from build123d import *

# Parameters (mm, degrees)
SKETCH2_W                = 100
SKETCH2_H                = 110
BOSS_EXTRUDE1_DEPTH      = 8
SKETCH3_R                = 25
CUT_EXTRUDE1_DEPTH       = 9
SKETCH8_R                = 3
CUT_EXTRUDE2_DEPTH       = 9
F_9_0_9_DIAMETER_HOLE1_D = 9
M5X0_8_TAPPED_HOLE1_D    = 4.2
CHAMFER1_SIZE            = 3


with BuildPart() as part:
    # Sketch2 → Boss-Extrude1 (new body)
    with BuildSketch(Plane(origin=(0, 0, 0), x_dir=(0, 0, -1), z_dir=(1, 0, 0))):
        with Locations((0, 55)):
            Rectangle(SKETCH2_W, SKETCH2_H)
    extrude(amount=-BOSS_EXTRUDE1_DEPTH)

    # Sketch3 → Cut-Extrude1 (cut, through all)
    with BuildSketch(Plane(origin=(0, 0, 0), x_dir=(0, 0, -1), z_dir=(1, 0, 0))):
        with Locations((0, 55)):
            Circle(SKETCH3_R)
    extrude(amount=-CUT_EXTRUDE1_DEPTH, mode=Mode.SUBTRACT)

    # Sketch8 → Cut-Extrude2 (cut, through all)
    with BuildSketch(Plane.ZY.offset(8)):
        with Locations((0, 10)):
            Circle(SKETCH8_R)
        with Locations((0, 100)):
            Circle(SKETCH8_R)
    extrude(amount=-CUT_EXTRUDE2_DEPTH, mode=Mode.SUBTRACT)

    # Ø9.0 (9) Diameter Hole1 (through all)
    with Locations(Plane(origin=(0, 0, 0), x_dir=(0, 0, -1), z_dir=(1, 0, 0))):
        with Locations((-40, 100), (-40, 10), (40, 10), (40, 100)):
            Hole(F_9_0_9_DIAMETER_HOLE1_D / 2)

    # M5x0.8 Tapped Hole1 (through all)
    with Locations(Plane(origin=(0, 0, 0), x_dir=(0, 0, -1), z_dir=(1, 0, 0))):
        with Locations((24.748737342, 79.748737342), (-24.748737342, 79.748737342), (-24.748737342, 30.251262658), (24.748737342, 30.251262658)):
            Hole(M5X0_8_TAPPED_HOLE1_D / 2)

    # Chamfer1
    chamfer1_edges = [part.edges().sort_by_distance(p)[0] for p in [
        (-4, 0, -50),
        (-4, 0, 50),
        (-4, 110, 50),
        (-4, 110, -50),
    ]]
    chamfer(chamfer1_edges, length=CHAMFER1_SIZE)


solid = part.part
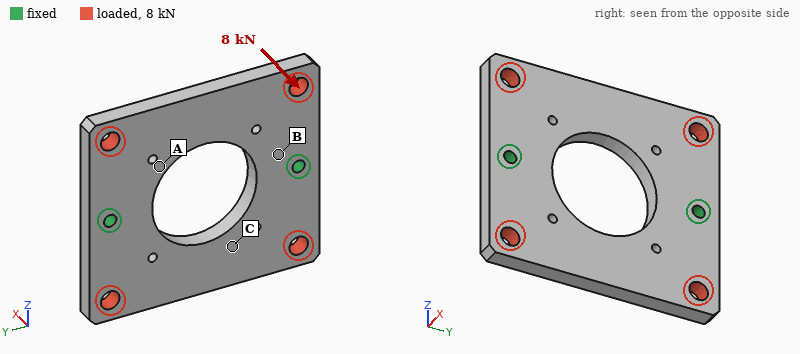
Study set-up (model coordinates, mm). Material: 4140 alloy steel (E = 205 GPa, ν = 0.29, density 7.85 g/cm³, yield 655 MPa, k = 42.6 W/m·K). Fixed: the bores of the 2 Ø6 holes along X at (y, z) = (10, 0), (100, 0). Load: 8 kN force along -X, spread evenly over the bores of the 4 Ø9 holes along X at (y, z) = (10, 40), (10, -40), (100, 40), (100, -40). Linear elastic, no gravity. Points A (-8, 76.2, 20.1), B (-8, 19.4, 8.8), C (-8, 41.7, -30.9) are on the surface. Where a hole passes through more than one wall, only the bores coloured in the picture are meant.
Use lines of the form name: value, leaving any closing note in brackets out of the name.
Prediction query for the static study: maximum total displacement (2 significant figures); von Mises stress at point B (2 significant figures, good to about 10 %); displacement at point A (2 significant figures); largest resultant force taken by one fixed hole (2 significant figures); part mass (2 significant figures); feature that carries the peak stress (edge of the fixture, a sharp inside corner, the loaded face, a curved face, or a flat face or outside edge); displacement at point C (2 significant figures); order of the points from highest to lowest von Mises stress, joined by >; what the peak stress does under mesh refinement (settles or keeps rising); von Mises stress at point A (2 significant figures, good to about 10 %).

maximum total displacement: 0.20 mm
von Mises stress at point B: 170 MPa
displacement at point A: 0.044 mm
largest resultant force taken by one fixed hole: 4.0 kN
part mass: 540 g
feature that carries the peak stress: edge of the fixture
displacement at point C: 0.087 mm
order of the points from highest to lowest von Mises stress, joined by >: B > A > C
what the peak stress does under mesh refinement: keeps rising
von Mises stress at point A: 81 MPa
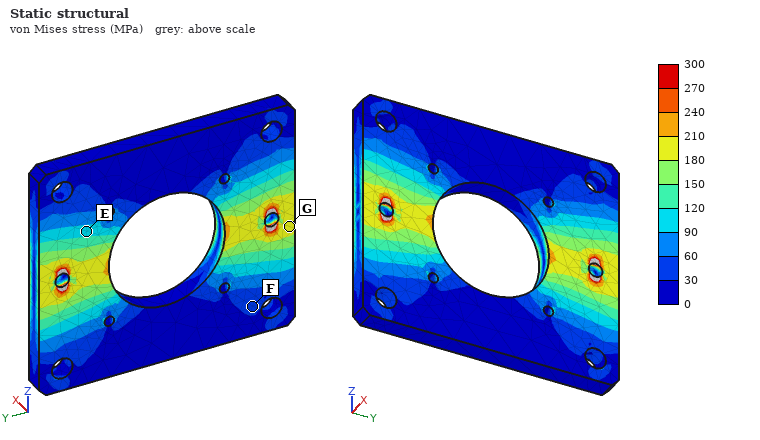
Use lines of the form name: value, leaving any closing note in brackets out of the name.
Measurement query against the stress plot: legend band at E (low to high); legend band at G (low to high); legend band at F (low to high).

legend band at E: 90 to 120 MPa
legend band at G: 180 to 210 MPa
legend band at F: 30 to 60 MPa
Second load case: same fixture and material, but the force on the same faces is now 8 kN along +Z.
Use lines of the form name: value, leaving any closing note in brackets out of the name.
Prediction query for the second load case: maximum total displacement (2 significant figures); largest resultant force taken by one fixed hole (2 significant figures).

maximum total displacement: 3.4 µm
largest resultant force taken by one fixed hole: 4.0 kN
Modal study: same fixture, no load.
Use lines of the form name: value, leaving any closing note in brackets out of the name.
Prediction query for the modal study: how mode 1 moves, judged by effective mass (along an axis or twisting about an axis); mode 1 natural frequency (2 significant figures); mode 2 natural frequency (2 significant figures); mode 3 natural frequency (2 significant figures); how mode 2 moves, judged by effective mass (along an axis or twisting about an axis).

how mode 1 moves, judged by effective mass: twisting about Y
mode 1 natural frequency: 1700 Hz
mode 2 natural frequency: 2000 Hz
mode 3 natural frequency: 3400 Hz
how mode 2 moves, judged by effective mass: along X
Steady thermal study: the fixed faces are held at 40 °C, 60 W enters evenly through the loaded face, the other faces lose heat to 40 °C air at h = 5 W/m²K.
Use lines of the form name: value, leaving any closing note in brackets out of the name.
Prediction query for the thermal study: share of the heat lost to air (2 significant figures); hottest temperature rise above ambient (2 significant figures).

share of the heat lost to air: 7.6 %
hottest temperature rise above ambient: 71 K
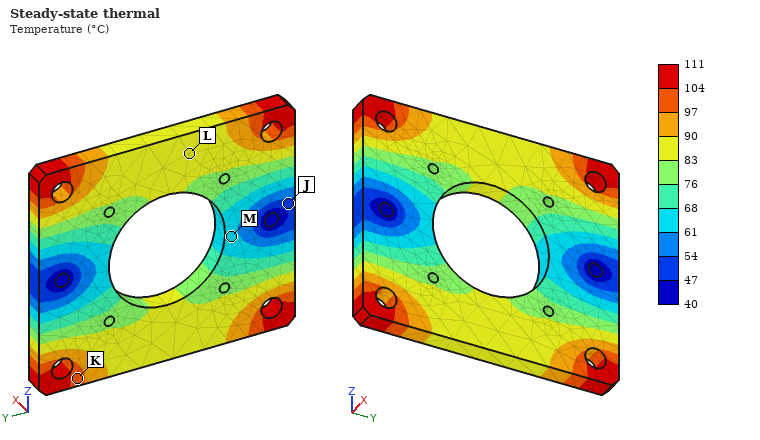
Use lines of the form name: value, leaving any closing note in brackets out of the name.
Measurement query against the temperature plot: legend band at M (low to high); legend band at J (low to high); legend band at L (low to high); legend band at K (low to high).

legend band at M: 61 to 68 °C
legend band at J: 47 to 54 °C
legend band at L: 83 to 90 °C
legend band at K: 97 to 104 °C
